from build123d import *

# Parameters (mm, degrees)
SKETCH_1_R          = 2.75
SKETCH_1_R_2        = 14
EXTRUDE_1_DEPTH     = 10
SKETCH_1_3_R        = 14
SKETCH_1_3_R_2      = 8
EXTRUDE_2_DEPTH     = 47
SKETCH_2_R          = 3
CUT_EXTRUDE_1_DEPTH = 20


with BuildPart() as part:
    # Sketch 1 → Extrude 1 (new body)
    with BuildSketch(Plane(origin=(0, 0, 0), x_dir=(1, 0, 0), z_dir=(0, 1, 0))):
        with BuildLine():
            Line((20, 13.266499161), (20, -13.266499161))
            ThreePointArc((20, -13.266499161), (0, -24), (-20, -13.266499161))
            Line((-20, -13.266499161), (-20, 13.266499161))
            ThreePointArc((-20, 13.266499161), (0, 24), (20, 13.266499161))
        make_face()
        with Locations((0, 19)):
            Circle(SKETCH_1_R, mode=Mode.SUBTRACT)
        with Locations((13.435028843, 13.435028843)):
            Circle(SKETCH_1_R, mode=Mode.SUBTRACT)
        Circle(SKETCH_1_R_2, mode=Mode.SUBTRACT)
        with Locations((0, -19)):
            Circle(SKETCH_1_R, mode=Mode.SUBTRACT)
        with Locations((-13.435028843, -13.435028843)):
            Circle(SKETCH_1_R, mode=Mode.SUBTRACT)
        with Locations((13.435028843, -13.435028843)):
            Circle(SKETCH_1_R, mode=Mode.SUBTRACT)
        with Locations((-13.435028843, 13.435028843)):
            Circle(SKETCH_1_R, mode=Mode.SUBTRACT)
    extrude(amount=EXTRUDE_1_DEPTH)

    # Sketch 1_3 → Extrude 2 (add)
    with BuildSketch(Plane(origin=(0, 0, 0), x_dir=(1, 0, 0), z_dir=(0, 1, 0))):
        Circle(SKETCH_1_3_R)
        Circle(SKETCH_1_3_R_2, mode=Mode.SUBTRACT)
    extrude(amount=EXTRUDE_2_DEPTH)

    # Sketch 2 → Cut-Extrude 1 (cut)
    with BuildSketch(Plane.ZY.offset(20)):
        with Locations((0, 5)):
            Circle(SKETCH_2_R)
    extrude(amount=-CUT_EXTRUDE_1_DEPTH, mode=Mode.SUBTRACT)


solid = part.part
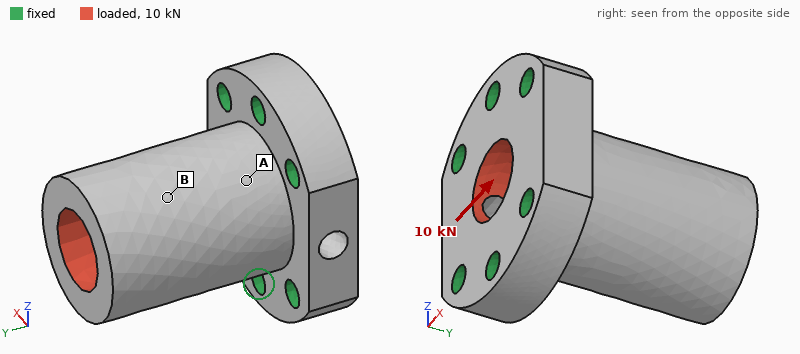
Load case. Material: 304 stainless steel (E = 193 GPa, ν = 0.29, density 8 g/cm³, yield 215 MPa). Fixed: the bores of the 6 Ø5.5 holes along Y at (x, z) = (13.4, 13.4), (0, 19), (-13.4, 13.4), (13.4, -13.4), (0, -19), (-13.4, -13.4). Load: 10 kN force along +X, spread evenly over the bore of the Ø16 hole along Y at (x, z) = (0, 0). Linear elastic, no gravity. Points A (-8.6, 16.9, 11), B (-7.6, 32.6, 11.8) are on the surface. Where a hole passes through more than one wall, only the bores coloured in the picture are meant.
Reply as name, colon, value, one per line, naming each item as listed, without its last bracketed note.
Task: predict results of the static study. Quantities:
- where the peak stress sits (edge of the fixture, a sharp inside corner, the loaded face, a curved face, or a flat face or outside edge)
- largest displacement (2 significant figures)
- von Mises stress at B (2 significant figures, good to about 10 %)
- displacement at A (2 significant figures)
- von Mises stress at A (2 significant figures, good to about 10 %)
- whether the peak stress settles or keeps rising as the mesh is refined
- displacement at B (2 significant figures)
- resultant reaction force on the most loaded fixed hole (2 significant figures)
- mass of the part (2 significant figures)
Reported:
where the peak stress sits: edge of the fixture
largest displacement: 31 µm
von Mises stress at B: 19 MPa
displacement at A: 7.7 µm
von Mises stress at A: 41 MPa
whether the peak stress settles or keeps rising as the mesh is refined: keeps rising
displacement at B: 20 µm
resultant reaction force on the most loaded fixed hole: 4.2 kN
mass of the part: 230 g
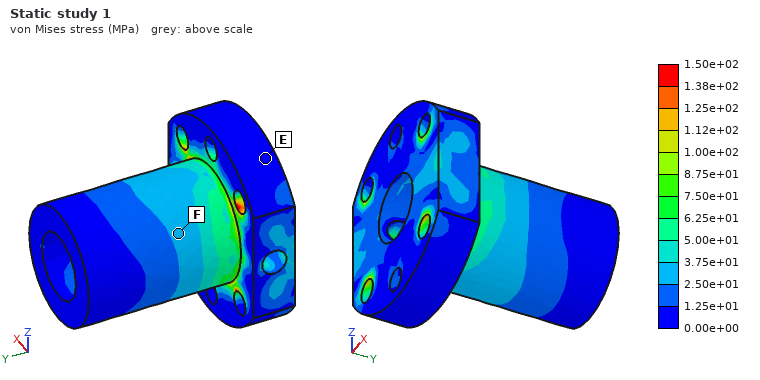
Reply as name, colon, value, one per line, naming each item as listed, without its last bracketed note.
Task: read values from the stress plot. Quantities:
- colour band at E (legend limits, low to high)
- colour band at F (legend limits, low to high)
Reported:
colour band at E: 0.00e+00 to 1.25e+01 MPa
colour band at F: 2.50e+01 to 3.75e+01 MPa
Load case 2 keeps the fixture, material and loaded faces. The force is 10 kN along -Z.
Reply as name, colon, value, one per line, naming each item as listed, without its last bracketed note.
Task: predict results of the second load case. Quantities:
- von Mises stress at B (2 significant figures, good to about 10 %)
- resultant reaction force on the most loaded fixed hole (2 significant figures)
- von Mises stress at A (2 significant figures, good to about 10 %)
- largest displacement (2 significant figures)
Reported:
von Mises stress at B: 15 MPa
resultant reaction force on the most loaded fixed hole: 3.5 kN
von Mises stress at A: 43 MPa
largest displacement: 26 µm
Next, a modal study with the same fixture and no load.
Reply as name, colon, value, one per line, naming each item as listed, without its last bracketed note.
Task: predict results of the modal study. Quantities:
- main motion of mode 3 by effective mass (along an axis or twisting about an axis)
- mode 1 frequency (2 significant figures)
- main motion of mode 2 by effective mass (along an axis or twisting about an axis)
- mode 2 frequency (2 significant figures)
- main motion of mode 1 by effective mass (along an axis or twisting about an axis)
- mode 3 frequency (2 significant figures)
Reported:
main motion of mode 3 by effective mass: twisting about Y
mode 1 frequency: 8700 Hz
main motion of mode 2 by effective mass: along Z
mode 2 frequency: 9400 Hz
main motion of mode 1 by effective mass: along X
mode 3 frequency: 19 kHz
